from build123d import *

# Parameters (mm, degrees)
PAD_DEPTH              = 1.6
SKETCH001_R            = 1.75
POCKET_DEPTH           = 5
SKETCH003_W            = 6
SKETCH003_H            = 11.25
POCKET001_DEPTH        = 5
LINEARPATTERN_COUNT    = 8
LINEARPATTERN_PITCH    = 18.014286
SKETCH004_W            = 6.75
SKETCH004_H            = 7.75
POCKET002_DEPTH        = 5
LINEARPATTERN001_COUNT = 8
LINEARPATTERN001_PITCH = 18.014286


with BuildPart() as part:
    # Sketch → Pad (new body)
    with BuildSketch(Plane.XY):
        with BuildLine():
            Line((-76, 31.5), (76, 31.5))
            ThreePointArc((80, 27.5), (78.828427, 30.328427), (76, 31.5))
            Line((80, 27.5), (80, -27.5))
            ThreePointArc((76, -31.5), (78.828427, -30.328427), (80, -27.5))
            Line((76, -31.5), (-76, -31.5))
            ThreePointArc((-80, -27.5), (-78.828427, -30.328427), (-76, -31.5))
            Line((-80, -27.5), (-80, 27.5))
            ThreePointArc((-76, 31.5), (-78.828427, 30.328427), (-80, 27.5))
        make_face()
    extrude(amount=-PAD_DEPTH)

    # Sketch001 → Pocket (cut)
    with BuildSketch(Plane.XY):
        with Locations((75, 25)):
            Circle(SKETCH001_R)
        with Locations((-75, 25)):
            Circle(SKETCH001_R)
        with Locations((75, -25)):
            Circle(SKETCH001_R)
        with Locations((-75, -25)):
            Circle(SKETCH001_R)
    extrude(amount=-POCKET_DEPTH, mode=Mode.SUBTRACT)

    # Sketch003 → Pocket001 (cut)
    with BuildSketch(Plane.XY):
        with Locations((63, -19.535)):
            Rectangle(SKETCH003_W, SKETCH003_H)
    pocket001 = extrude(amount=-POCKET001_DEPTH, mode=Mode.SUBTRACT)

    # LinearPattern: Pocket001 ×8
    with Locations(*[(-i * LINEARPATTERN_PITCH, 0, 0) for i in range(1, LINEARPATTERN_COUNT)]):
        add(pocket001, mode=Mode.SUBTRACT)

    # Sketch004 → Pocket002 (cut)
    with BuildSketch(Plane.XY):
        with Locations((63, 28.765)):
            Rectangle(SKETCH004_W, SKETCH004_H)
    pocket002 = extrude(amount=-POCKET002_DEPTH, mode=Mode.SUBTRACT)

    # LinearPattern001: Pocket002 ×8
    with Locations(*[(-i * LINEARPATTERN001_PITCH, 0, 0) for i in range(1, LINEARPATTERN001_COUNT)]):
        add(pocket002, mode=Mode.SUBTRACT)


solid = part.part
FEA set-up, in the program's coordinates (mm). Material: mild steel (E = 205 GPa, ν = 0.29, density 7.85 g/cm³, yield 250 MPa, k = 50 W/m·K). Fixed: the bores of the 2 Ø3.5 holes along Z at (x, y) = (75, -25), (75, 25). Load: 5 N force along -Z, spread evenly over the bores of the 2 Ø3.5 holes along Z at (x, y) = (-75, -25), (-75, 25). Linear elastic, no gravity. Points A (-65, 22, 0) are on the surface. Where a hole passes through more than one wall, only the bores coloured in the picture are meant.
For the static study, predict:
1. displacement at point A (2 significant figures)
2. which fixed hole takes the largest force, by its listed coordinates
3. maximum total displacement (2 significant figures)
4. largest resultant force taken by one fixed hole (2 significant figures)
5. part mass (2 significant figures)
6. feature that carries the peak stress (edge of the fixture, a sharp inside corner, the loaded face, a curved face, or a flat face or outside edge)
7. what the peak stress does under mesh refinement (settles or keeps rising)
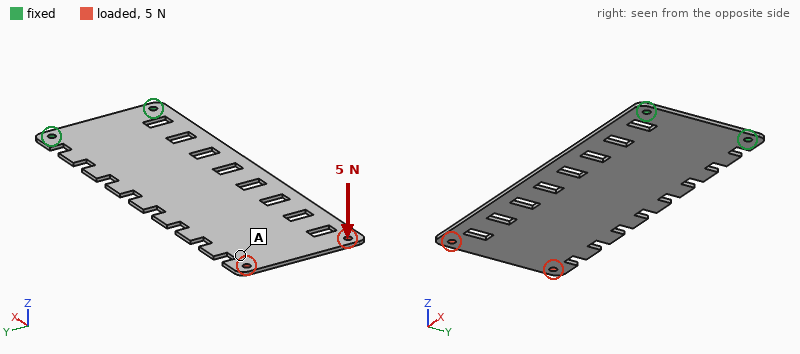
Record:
1.6 mm
(75, -25)
1.9 mm
2.7 N
110 g
edge of the fixture
keeps rising
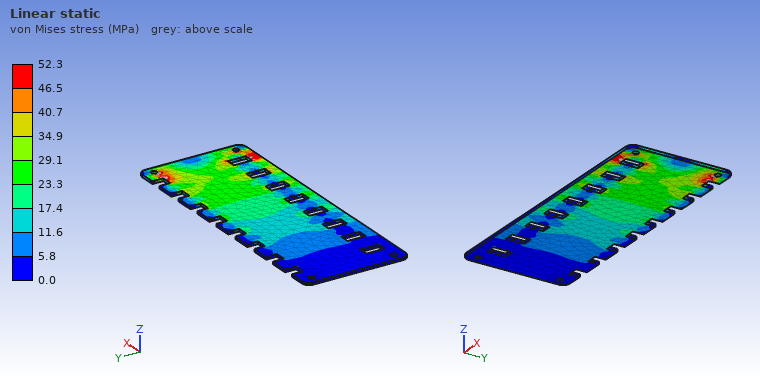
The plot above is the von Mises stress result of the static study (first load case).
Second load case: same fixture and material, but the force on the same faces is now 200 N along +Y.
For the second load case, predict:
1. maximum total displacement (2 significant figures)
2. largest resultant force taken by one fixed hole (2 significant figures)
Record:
73 µm
620 N
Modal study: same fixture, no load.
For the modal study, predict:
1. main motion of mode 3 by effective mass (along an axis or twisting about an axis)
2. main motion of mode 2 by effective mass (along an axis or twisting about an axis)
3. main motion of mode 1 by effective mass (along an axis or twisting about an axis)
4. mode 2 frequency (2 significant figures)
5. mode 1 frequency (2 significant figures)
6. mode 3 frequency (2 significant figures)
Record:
along Z
twisting about X
along Z
280 Hz
48 Hz
310 Hz
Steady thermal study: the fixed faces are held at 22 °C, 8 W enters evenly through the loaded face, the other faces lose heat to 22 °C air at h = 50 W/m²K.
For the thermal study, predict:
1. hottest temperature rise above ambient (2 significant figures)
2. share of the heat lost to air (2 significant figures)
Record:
65 K
100 %
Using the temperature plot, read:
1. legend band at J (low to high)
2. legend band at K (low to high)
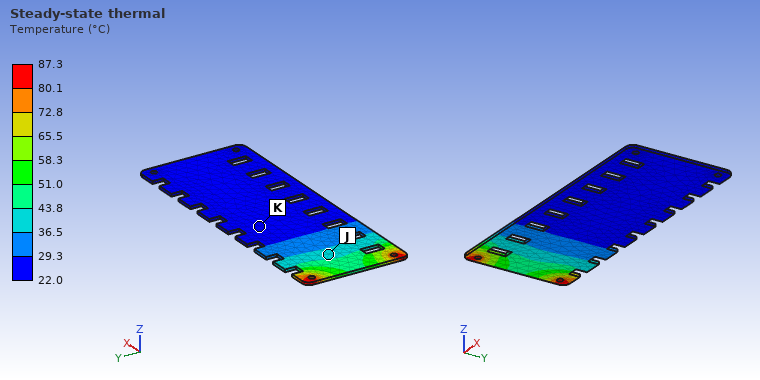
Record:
36.5 to 43.8 °C
22.0 to 29.3 °C
